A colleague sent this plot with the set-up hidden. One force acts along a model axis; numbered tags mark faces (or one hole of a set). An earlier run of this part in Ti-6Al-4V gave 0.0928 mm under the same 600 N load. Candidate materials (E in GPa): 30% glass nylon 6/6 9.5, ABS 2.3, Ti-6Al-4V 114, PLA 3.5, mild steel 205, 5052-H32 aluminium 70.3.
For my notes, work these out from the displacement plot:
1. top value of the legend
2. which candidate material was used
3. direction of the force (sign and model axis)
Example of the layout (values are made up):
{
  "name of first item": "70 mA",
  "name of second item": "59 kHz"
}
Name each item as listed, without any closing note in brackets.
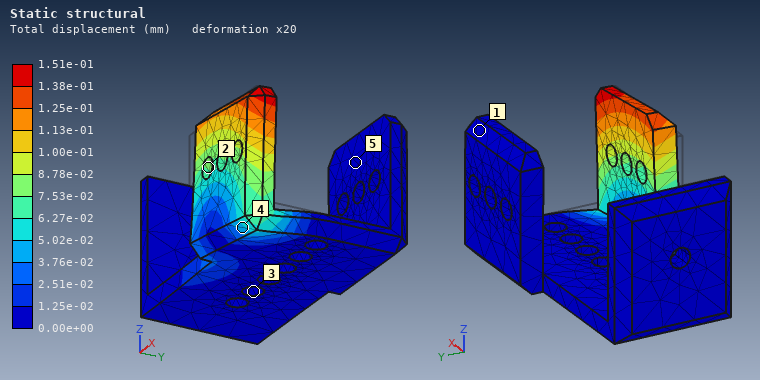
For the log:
{
  "top value of the legend": "1.51e-01 mm",
  "which candidate material was used": "5052-H32 aluminium",
  "direction of the force": "+X"
}
